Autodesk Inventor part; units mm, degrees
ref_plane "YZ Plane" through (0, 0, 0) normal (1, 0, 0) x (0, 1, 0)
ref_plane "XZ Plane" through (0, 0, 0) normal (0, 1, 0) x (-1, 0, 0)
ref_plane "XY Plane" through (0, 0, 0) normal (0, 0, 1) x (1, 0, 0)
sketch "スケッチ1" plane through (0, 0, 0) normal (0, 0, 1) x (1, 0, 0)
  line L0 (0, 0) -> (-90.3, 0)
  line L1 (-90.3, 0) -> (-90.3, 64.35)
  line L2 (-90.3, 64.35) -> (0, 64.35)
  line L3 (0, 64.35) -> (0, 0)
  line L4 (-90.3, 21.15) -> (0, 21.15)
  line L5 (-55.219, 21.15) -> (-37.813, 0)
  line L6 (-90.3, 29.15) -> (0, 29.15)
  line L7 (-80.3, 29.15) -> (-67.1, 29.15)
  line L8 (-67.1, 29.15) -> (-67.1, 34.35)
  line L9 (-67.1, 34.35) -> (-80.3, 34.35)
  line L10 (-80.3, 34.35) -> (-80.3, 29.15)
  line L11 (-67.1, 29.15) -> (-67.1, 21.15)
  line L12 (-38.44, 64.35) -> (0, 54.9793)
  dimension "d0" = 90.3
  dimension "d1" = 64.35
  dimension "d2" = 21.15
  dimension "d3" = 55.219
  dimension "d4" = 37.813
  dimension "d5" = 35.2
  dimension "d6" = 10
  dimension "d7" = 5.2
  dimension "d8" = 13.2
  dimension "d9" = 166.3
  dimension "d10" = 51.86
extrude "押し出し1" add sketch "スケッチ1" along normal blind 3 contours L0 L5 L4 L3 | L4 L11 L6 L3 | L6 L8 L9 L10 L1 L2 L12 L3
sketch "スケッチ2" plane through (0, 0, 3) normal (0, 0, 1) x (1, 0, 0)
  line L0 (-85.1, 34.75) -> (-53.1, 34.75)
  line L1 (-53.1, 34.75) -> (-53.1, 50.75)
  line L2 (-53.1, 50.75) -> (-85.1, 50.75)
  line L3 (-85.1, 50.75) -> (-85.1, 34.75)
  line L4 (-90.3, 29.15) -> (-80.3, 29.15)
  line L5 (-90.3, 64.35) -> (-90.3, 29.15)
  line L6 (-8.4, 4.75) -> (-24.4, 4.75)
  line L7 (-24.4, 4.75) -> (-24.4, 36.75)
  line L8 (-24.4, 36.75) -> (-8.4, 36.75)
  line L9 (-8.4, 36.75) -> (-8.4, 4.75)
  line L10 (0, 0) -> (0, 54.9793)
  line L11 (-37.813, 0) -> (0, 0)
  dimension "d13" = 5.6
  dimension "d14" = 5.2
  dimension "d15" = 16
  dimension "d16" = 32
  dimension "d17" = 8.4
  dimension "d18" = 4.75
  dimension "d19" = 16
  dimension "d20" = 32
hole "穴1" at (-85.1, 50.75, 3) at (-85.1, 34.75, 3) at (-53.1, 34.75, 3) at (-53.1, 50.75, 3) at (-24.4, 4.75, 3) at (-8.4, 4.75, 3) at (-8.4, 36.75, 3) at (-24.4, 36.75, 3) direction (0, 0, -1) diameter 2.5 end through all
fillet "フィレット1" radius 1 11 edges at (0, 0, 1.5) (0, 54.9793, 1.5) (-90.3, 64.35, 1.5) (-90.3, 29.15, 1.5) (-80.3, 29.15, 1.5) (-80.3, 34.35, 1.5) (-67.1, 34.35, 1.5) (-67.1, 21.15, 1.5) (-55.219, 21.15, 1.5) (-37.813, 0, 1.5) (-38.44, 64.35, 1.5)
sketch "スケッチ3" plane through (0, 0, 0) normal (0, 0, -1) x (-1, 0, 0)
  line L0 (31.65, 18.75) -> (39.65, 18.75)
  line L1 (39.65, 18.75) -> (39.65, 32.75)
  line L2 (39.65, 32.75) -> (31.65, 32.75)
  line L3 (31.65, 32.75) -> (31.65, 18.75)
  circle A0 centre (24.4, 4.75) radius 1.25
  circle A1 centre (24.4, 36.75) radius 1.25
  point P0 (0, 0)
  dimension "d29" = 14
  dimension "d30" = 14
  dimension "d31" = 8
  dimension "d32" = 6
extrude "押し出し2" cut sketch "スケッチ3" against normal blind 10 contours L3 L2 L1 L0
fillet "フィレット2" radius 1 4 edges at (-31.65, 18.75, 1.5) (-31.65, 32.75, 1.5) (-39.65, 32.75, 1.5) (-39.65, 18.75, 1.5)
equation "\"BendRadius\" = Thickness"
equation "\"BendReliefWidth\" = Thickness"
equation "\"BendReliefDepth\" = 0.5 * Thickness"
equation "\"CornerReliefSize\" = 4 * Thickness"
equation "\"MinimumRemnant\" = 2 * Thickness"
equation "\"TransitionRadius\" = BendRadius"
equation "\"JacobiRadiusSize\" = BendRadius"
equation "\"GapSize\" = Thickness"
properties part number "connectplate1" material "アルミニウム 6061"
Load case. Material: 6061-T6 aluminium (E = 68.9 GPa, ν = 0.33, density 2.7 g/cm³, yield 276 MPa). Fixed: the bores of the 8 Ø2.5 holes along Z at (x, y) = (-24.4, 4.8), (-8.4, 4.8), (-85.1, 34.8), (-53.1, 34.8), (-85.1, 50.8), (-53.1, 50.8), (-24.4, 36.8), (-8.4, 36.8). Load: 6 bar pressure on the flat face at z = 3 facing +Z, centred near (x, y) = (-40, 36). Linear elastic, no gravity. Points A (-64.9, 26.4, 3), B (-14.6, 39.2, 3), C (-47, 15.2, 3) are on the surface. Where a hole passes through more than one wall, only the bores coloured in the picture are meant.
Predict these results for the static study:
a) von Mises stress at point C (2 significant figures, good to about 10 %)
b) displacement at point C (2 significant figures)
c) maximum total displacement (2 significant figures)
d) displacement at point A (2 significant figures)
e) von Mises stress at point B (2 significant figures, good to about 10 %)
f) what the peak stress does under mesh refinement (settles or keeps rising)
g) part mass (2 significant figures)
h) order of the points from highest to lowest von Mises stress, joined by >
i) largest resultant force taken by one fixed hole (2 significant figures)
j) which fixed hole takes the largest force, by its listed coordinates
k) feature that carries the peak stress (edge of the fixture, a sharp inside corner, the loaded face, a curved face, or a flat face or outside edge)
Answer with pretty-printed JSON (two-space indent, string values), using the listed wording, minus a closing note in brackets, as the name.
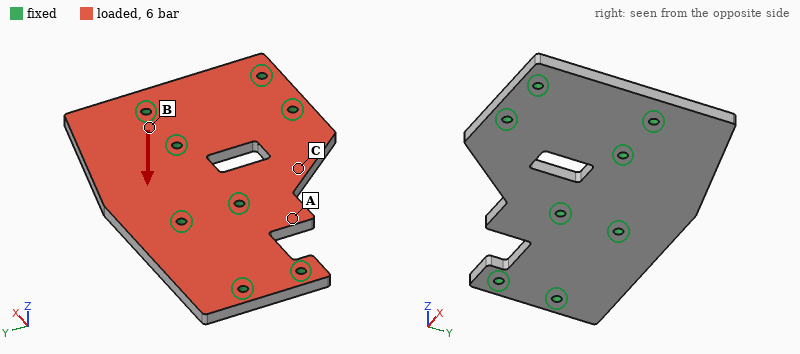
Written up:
{
  "von Mises stress at point C": "25 MPa",
  "displacement at point C": "0.045 mm",
  "maximum total displacement": "0.10 mm",
  "displacement at point A": "0.026 mm",
  "von Mises stress at point B": "48 MPa",
  "what the peak stress does under mesh refinement": "keeps rising",
  "part mass": "35 g",
  "order of the points from highest to lowest von Mises stress, joined by >": "B > C > A",
  "largest resultant force taken by one fixed hole": "510 N",
  "which fixed hole takes the largest force, by its listed coordinates": "(-53.1, 50.8)",
  "feature that carries the peak stress": "edge of the fixture"
}
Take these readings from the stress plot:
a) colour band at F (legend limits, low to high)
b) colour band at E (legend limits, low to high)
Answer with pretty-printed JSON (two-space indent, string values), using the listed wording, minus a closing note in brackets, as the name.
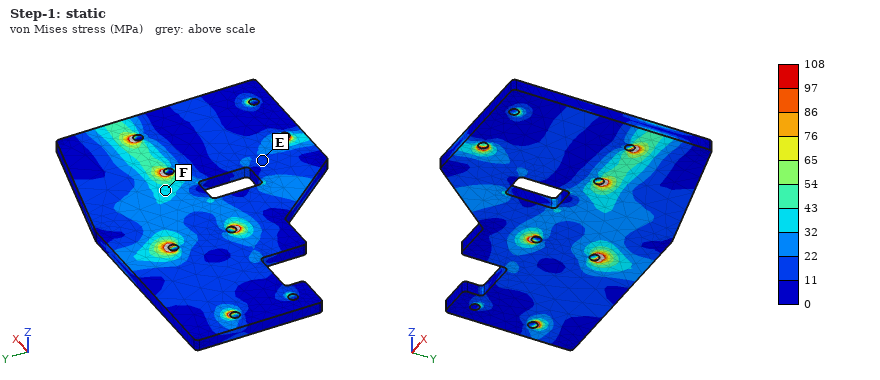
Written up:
{
  "colour band at F": "32 to 43 MPa",
  "colour band at E": "11 to 22 MPa"
}
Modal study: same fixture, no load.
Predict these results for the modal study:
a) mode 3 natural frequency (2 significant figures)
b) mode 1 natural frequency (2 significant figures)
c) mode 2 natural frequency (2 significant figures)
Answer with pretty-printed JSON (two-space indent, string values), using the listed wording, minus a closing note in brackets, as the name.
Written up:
{
  "mode 3 natural frequency": "9200 Hz",
  "mode 1 natural frequency": "5500 Hz",
  "mode 2 natural frequency": "7800 Hz"
}
